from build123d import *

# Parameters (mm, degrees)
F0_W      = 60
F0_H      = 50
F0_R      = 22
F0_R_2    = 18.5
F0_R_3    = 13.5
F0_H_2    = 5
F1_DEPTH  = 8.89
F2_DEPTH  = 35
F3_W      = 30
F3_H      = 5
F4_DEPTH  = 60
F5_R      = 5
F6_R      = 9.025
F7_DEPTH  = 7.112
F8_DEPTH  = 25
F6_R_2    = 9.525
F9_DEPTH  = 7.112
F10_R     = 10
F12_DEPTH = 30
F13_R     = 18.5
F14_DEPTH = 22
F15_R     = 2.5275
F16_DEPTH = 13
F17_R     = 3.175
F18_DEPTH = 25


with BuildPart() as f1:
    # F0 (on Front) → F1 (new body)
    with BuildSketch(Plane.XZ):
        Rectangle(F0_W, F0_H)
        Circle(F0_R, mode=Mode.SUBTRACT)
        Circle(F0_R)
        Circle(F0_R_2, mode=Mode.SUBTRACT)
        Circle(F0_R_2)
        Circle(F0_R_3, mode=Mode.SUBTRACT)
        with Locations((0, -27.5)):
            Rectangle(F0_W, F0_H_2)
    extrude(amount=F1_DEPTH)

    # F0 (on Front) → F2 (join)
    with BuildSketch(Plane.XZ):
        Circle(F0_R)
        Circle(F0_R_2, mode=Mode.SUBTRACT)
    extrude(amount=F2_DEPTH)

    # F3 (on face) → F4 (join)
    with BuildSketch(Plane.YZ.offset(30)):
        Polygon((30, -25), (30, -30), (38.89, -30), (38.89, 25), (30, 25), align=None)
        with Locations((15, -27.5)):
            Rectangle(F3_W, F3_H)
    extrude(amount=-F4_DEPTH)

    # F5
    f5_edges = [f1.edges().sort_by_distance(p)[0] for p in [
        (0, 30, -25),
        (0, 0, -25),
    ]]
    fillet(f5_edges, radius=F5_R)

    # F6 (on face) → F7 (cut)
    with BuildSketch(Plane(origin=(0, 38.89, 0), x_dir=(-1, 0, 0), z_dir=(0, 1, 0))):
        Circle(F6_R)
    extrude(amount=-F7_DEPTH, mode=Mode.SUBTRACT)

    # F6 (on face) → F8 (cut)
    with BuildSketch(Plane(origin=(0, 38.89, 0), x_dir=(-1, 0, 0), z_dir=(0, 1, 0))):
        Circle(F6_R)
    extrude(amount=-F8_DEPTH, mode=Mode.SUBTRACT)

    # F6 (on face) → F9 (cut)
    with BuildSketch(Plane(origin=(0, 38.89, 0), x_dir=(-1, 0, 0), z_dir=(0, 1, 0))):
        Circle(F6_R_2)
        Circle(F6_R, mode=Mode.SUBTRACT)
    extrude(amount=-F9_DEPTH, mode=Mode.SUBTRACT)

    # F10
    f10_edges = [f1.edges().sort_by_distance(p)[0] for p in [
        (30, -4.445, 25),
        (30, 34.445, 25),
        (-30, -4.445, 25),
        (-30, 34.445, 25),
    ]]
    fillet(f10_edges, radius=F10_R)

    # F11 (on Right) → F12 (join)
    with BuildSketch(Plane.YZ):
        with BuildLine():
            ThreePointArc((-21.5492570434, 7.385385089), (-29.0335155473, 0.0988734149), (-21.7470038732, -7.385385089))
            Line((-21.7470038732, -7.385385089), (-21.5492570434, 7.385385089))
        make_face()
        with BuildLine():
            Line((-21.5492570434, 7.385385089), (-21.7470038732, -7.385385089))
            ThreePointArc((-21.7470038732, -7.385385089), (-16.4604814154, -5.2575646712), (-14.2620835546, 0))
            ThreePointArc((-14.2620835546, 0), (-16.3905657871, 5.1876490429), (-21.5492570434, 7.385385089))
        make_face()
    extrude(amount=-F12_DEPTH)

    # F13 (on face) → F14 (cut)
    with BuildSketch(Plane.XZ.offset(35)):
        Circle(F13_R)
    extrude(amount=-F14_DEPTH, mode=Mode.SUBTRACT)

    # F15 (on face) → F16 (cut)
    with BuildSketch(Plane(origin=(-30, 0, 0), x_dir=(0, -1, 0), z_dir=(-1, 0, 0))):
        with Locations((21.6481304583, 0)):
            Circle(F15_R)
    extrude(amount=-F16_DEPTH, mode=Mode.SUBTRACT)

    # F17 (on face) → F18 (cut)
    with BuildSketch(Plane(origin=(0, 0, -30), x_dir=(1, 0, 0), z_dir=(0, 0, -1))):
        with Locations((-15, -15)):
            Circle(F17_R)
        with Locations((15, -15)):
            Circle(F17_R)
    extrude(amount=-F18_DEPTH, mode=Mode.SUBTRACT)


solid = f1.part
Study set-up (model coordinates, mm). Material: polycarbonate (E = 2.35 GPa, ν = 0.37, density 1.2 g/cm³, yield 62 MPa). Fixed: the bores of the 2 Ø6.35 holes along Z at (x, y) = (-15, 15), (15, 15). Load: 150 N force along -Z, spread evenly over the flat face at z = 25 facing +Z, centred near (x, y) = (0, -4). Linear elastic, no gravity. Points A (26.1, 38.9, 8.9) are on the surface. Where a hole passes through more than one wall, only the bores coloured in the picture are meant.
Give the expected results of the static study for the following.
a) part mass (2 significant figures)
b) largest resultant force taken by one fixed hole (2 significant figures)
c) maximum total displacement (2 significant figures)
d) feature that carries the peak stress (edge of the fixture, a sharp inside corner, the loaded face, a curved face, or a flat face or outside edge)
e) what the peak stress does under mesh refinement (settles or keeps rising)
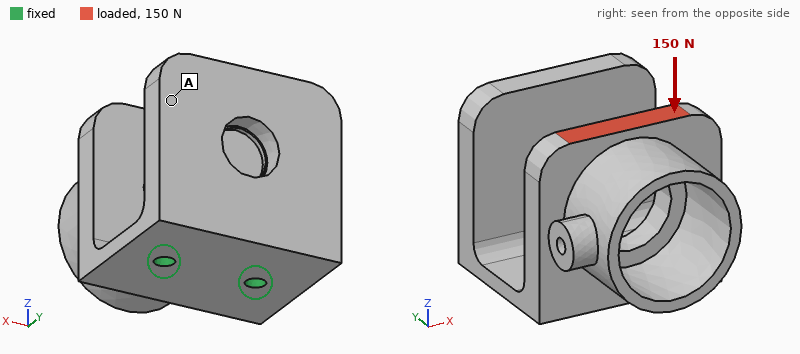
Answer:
87 g
75 N
1.1 mm
edge of the fixture
keeps rising
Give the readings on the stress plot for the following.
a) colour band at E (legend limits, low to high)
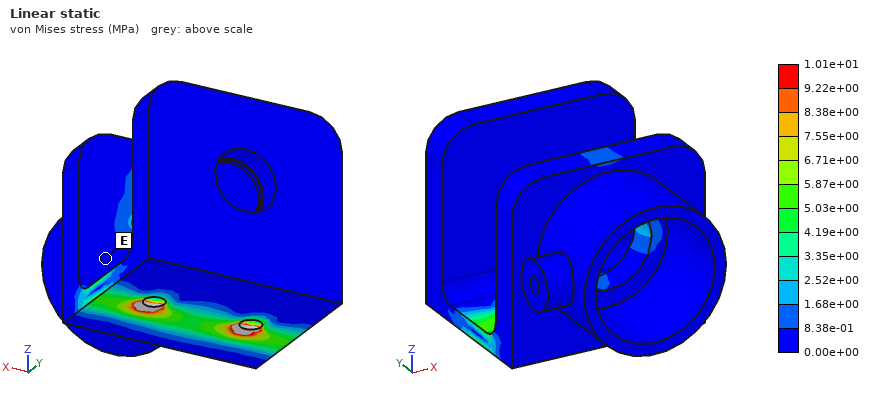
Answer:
0.00e+00 to 8.38e-01 MPa
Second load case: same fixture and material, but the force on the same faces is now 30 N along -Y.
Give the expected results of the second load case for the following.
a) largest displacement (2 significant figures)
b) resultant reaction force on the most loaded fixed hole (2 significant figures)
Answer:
1.1 mm
15 N
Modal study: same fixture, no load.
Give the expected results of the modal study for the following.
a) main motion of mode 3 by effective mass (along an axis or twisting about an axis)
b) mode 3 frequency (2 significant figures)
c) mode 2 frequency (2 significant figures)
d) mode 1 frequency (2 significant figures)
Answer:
along X
580 Hz
280 Hz
210 Hz
